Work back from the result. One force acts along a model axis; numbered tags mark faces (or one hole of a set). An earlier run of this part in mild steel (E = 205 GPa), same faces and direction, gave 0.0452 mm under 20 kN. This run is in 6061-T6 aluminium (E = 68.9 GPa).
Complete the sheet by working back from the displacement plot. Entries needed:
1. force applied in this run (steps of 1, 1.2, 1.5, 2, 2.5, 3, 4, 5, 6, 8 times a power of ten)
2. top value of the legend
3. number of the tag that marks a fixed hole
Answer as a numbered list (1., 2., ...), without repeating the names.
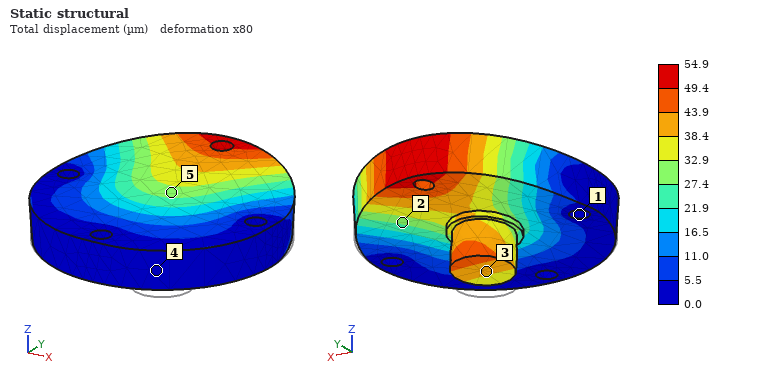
1. 8 kN
2. 54.9 µm
3. 1
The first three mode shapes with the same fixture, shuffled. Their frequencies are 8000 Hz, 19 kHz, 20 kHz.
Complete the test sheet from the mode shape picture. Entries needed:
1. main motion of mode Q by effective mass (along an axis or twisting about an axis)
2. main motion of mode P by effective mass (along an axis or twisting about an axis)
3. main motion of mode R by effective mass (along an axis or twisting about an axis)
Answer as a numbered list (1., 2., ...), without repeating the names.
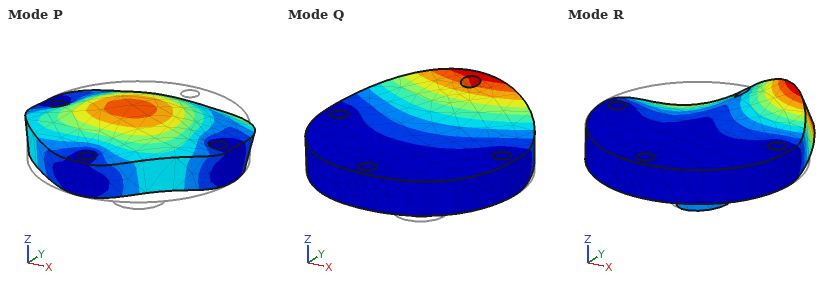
1. along Z
2. along Z
3. twisting about Y
